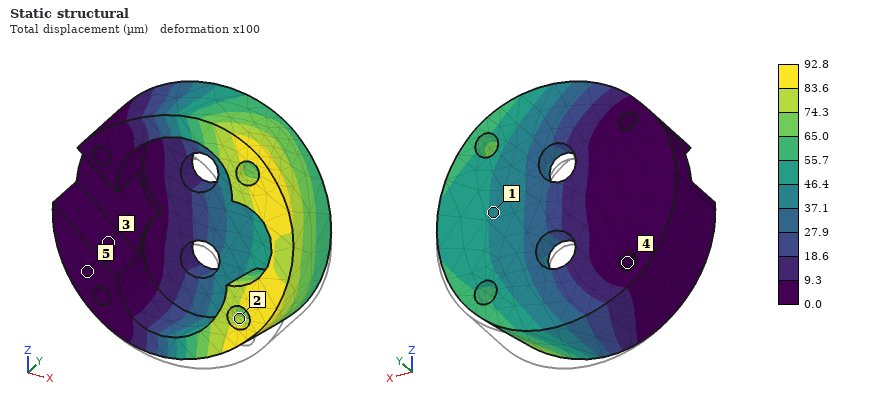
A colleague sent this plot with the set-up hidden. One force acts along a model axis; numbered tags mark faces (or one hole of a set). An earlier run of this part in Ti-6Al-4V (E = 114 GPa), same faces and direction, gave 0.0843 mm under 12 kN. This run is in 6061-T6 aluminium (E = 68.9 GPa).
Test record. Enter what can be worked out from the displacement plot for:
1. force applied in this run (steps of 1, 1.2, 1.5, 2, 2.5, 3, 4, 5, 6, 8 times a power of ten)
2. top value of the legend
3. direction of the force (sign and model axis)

8 kN
92.8 µm
+Z
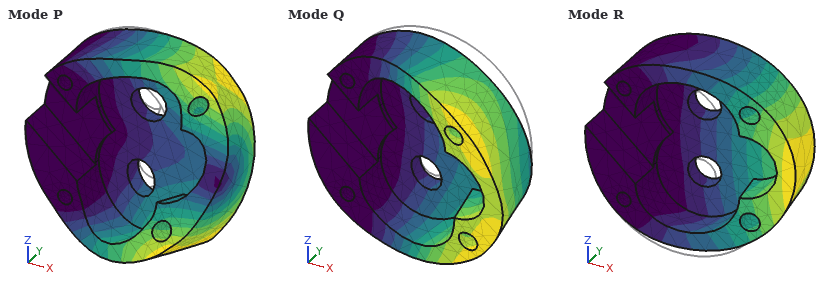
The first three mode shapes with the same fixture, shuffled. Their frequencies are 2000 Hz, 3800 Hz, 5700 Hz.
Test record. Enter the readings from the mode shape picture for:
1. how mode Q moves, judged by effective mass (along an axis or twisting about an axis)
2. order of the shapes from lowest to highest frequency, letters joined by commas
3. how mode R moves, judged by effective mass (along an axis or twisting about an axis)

along Z
R, Q, P
along Y
